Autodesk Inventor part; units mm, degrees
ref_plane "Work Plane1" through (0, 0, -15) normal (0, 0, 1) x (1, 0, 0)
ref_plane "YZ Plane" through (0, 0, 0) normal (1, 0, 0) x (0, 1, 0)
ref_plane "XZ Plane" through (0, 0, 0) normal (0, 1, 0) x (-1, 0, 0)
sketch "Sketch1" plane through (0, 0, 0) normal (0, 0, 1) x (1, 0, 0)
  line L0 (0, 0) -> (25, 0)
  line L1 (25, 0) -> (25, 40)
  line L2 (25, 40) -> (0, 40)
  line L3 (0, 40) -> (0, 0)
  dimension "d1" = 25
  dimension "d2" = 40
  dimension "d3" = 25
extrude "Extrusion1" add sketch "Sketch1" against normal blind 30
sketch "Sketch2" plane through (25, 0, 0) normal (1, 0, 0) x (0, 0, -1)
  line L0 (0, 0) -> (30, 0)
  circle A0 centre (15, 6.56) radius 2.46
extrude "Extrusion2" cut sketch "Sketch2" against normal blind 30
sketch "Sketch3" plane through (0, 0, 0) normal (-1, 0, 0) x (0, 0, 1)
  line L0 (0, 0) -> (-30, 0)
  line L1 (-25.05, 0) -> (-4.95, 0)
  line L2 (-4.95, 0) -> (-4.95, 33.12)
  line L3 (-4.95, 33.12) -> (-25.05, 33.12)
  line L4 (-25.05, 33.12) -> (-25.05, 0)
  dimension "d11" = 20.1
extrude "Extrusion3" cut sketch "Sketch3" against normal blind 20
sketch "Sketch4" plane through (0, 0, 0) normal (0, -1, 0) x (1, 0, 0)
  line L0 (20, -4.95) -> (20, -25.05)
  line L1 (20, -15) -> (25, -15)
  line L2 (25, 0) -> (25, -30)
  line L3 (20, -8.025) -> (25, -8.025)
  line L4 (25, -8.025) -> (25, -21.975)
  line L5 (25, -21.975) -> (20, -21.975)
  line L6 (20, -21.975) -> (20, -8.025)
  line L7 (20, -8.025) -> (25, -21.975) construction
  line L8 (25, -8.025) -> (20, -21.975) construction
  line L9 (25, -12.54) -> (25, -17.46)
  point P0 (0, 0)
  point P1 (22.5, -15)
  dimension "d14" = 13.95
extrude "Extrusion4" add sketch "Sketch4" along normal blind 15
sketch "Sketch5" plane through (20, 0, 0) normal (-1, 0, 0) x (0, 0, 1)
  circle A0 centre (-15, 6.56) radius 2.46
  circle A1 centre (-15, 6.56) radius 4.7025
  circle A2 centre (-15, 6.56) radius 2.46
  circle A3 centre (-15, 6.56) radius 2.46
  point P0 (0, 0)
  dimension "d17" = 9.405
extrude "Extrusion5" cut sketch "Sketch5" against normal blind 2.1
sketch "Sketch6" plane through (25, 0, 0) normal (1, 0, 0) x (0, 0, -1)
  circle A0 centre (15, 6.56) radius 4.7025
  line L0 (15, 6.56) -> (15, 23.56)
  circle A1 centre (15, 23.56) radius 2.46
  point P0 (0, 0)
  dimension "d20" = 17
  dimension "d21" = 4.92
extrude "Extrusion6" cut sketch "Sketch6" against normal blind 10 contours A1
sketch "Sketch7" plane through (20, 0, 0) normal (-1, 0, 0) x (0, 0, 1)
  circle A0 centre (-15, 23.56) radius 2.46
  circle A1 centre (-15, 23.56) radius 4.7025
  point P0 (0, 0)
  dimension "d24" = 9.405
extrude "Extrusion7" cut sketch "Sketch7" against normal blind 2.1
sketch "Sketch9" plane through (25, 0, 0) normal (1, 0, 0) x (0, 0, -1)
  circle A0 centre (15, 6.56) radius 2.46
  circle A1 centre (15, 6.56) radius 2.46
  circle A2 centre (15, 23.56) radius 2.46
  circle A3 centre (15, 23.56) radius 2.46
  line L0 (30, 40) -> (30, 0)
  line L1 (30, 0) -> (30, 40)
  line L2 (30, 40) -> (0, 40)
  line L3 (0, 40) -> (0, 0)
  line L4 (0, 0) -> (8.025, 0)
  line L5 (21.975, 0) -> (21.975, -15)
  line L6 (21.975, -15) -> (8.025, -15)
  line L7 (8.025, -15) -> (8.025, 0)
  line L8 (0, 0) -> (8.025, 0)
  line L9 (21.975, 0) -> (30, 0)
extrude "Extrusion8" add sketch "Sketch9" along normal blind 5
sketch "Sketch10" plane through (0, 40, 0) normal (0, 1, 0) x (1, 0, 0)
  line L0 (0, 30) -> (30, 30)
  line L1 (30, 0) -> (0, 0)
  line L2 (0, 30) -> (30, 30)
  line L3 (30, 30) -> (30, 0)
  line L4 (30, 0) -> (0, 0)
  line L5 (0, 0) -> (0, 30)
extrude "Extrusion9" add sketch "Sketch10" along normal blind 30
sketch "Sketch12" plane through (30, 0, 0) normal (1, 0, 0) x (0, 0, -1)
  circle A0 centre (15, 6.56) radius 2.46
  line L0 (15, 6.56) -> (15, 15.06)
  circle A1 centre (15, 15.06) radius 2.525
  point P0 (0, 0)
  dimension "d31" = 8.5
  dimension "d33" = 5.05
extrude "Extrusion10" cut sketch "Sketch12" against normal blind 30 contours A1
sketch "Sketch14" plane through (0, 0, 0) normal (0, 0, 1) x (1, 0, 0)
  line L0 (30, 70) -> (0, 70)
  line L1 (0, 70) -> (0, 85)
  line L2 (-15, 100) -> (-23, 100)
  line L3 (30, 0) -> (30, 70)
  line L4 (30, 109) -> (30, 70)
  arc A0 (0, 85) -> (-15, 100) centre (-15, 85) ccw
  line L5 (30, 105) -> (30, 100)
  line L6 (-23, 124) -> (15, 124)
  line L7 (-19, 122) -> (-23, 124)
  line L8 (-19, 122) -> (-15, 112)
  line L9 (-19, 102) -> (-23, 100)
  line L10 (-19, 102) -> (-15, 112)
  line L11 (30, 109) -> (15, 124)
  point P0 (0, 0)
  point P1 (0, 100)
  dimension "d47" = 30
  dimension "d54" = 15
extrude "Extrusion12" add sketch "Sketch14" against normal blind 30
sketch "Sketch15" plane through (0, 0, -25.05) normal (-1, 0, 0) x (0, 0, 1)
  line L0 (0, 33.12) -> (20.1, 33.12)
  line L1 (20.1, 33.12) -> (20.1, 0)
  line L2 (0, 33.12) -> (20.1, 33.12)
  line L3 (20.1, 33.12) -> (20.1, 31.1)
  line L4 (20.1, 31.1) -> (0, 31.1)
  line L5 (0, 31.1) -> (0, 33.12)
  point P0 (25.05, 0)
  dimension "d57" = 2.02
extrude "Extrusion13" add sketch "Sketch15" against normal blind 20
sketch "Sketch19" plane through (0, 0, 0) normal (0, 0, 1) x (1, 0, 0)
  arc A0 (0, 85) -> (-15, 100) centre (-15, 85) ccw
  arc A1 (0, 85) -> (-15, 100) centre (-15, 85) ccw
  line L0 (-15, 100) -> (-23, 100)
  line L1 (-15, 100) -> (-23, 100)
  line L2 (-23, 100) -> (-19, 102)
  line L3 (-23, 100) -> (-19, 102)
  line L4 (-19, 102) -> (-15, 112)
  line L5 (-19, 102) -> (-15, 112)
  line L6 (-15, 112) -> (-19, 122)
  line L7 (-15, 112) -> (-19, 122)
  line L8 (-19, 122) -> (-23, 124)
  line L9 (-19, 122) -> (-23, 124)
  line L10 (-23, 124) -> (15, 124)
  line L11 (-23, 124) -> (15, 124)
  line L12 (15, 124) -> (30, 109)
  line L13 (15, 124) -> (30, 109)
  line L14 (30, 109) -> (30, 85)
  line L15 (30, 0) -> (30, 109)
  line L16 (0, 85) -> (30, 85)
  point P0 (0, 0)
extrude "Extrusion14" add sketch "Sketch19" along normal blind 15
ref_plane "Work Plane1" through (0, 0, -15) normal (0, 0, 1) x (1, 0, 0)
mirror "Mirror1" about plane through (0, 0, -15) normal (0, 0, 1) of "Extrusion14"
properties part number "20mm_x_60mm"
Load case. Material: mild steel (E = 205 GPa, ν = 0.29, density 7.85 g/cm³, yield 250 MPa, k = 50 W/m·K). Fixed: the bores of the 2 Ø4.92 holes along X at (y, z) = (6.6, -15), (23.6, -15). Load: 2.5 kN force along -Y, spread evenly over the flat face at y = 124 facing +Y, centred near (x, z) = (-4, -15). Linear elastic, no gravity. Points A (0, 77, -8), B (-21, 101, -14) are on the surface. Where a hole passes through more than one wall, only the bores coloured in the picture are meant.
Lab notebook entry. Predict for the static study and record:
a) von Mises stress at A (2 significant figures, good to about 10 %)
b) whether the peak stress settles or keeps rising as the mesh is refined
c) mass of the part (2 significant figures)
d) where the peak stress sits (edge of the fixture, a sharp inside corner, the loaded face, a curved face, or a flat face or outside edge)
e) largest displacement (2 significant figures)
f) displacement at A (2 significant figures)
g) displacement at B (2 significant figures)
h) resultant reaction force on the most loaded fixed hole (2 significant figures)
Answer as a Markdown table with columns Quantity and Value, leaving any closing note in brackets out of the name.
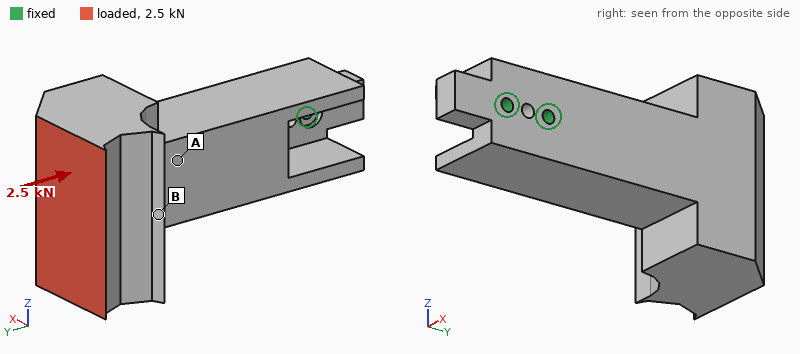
| Quantity | Value |
|---|---|
| von Mises stress at A | 14 MPa |
| whether the peak stress settles or keeps rising as the mesh is refined | keeps rising |
| mass of the part | 1.2 kg |
| where the peak stress sits | edge of the fixture |
| largest displacement | 78 µm |
| displacement at A | 37 µm |
| displacement at B | 61 µm |
| resultant reaction force on the most loaded fixed hole | 3.4 kN |
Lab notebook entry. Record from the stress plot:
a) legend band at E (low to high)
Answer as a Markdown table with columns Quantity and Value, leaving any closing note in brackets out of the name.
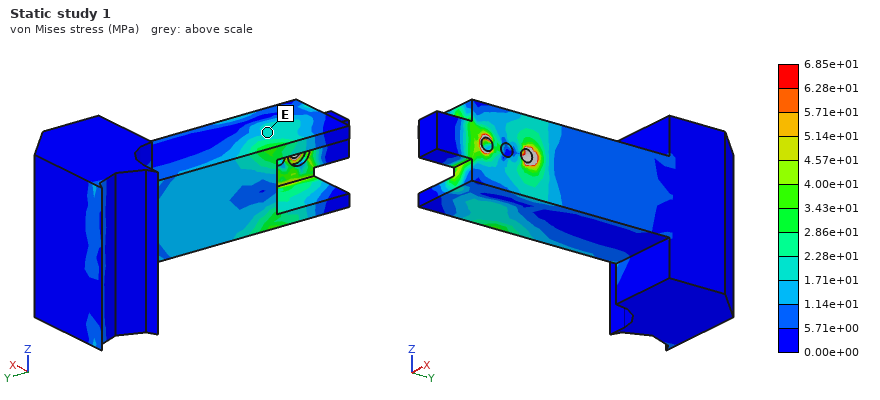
| Quantity | Value |
|---|---|
| legend band at E | 1.71e+01 to 2.28e+01 MPa |
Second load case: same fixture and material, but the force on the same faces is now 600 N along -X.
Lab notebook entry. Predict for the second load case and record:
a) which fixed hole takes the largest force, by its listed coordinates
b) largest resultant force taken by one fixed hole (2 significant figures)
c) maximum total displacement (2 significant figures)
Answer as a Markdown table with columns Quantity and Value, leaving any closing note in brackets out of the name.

| Quantity | Value |
|---|---|
| which fixed hole takes the largest force, by its listed coordinates | (23.6, -15) |
| largest resultant force taken by one fixed hole | 3.0 kN |
| maximum total displacement | 64 µm |
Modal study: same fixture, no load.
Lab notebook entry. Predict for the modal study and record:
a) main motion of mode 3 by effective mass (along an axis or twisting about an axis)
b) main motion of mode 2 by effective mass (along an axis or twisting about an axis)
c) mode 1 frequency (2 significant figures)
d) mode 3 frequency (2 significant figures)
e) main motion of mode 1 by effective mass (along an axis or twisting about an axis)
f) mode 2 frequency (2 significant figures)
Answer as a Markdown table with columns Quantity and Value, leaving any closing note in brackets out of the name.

| Quantity | Value |
|---|---|
| main motion of mode 3 by effective mass | twisting about Y |
| main motion of mode 2 by effective mass | along Z |
| mode 1 frequency | 690 Hz |
| mode 3 frequency | 1800 Hz |
| main motion of mode 1 by effective mass | along X |
| mode 2 frequency | 800 Hz |
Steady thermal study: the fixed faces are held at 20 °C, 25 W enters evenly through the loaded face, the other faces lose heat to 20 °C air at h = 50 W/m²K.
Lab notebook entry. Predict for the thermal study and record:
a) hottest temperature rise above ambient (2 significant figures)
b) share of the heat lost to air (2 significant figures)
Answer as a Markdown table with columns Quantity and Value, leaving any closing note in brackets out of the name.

| Quantity | Value |
|---|---|
| hottest temperature rise above ambient | 32 K |
| share of the heat lost to air | 68 % |
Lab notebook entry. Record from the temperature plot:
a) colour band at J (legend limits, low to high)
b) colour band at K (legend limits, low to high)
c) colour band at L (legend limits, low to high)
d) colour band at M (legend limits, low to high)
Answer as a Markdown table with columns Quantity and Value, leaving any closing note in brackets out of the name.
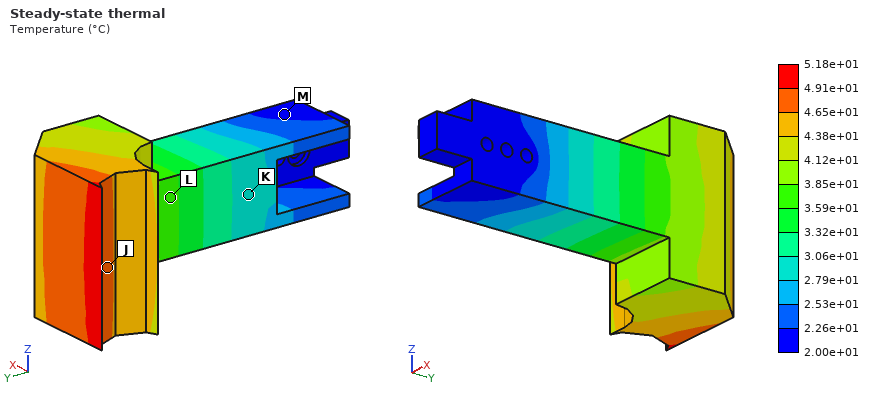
| Quantity | Value |
|---|---|
| colour band at J | 4.65e+01 to 4.91e+01 °C |
| colour band at K | 2.79e+01 to 3.06e+01 °C |
| colour band at L | 3.59e+01 to 3.85e+01 °C |
| colour band at M | 2.00e+01 to 2.26e+01 °C |
